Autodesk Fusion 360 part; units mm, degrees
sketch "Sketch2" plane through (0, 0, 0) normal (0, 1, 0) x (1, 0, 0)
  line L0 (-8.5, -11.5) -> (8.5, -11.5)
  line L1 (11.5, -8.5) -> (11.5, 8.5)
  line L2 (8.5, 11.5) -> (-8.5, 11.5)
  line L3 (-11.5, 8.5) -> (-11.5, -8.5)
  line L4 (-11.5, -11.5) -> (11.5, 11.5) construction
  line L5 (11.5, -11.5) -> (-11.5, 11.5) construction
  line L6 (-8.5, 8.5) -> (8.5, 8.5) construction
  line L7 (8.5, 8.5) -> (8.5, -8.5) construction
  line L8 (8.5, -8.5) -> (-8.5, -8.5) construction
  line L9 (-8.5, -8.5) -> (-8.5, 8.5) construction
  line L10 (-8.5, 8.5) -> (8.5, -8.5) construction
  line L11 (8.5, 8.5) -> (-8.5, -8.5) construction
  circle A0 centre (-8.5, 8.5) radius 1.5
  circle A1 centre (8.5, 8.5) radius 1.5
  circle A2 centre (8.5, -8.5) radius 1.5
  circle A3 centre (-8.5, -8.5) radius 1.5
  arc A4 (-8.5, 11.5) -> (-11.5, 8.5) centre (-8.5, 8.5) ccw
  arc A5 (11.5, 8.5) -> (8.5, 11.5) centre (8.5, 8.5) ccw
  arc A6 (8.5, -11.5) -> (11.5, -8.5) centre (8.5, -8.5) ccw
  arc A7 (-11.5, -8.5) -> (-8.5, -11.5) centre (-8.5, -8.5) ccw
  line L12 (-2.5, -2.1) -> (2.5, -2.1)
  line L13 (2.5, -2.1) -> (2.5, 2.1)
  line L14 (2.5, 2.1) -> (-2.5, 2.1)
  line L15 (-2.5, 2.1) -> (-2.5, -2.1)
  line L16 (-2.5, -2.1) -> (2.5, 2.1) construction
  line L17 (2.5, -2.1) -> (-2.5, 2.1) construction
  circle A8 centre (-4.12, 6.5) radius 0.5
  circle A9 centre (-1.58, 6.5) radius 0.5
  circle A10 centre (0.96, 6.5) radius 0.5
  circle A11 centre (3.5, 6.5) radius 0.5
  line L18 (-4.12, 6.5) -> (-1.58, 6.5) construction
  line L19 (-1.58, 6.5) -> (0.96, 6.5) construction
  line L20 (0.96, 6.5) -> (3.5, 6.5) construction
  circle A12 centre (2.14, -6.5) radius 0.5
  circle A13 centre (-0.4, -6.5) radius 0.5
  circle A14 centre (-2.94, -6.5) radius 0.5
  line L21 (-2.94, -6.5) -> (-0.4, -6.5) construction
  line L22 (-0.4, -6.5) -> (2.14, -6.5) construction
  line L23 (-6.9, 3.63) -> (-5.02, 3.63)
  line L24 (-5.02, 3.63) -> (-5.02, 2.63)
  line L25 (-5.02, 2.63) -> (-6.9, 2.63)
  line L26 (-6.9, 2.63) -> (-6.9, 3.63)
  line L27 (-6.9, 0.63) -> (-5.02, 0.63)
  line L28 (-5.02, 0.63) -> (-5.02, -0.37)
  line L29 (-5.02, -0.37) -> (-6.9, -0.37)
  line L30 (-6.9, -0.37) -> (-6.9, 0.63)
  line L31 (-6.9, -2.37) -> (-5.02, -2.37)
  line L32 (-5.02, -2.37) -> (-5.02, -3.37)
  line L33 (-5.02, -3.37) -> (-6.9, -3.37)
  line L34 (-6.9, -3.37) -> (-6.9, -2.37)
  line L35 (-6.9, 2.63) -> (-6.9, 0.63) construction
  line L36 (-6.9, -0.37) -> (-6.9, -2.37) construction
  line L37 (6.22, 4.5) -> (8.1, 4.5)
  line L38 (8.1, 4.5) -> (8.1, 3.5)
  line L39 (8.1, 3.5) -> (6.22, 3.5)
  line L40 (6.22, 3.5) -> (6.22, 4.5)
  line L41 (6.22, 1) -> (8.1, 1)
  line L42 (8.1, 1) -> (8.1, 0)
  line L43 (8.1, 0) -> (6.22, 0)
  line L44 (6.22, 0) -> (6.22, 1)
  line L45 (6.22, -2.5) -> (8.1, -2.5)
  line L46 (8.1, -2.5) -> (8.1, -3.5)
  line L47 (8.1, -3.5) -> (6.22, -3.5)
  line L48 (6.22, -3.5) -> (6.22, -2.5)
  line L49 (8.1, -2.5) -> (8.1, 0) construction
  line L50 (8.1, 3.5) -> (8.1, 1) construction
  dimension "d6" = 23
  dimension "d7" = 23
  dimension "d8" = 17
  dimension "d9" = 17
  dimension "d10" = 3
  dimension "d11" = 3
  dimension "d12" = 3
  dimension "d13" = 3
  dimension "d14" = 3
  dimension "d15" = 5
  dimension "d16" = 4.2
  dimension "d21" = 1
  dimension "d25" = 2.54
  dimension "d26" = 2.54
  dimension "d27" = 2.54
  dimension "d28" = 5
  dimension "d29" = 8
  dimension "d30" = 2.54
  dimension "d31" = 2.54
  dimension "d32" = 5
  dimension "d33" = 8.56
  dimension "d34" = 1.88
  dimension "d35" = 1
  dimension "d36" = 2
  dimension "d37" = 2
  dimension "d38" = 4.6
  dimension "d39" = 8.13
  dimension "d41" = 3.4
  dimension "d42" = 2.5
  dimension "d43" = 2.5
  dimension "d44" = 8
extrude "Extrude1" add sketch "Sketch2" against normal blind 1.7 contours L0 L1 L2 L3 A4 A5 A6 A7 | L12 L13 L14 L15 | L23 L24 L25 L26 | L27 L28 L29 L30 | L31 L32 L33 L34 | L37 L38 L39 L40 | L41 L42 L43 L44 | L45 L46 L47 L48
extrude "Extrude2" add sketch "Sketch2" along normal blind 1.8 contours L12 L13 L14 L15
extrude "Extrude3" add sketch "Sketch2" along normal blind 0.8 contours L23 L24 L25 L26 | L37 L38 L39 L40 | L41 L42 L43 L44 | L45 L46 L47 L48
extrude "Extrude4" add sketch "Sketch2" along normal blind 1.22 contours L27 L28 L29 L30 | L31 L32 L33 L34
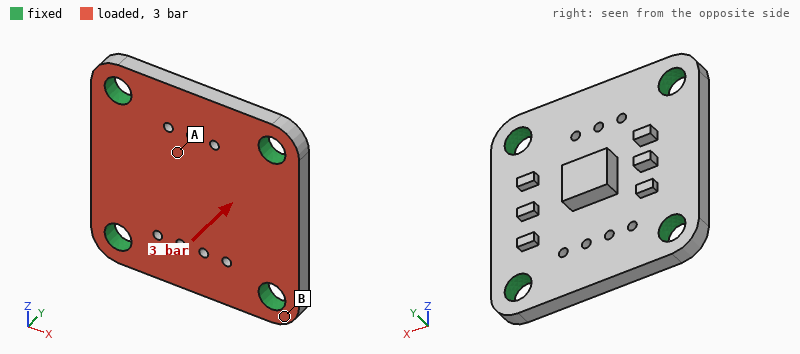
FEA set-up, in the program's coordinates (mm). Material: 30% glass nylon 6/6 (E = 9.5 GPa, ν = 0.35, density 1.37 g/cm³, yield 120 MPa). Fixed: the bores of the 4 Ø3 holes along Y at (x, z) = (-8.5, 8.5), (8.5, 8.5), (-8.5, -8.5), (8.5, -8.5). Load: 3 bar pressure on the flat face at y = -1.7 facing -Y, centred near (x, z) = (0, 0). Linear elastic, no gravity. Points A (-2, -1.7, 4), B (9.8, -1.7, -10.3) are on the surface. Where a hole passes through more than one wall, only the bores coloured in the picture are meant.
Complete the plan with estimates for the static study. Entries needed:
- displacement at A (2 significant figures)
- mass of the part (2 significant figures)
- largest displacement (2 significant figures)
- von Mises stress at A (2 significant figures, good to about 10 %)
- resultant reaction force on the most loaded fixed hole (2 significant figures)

21 µm
1.2 g
24 µm
5.6 MPa
37 N
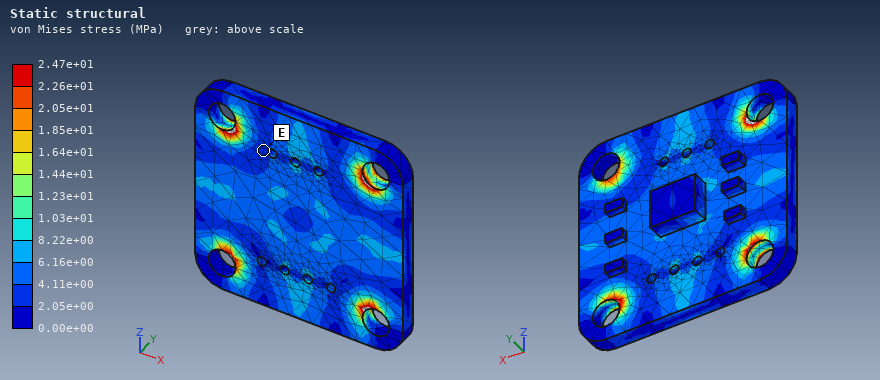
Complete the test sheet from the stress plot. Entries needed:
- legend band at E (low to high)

2.05e+00 to 4.11e+00 MPa
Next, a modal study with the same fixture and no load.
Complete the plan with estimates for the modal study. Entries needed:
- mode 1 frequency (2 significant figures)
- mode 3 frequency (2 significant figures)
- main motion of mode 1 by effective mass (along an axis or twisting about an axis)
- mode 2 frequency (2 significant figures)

13 kHz
20 kHz
along Y
20 kHz
